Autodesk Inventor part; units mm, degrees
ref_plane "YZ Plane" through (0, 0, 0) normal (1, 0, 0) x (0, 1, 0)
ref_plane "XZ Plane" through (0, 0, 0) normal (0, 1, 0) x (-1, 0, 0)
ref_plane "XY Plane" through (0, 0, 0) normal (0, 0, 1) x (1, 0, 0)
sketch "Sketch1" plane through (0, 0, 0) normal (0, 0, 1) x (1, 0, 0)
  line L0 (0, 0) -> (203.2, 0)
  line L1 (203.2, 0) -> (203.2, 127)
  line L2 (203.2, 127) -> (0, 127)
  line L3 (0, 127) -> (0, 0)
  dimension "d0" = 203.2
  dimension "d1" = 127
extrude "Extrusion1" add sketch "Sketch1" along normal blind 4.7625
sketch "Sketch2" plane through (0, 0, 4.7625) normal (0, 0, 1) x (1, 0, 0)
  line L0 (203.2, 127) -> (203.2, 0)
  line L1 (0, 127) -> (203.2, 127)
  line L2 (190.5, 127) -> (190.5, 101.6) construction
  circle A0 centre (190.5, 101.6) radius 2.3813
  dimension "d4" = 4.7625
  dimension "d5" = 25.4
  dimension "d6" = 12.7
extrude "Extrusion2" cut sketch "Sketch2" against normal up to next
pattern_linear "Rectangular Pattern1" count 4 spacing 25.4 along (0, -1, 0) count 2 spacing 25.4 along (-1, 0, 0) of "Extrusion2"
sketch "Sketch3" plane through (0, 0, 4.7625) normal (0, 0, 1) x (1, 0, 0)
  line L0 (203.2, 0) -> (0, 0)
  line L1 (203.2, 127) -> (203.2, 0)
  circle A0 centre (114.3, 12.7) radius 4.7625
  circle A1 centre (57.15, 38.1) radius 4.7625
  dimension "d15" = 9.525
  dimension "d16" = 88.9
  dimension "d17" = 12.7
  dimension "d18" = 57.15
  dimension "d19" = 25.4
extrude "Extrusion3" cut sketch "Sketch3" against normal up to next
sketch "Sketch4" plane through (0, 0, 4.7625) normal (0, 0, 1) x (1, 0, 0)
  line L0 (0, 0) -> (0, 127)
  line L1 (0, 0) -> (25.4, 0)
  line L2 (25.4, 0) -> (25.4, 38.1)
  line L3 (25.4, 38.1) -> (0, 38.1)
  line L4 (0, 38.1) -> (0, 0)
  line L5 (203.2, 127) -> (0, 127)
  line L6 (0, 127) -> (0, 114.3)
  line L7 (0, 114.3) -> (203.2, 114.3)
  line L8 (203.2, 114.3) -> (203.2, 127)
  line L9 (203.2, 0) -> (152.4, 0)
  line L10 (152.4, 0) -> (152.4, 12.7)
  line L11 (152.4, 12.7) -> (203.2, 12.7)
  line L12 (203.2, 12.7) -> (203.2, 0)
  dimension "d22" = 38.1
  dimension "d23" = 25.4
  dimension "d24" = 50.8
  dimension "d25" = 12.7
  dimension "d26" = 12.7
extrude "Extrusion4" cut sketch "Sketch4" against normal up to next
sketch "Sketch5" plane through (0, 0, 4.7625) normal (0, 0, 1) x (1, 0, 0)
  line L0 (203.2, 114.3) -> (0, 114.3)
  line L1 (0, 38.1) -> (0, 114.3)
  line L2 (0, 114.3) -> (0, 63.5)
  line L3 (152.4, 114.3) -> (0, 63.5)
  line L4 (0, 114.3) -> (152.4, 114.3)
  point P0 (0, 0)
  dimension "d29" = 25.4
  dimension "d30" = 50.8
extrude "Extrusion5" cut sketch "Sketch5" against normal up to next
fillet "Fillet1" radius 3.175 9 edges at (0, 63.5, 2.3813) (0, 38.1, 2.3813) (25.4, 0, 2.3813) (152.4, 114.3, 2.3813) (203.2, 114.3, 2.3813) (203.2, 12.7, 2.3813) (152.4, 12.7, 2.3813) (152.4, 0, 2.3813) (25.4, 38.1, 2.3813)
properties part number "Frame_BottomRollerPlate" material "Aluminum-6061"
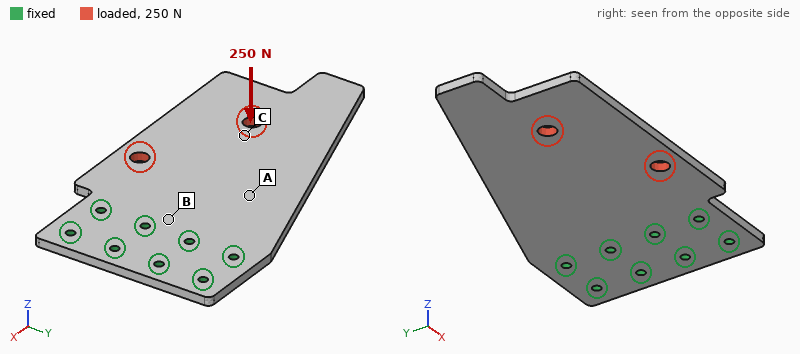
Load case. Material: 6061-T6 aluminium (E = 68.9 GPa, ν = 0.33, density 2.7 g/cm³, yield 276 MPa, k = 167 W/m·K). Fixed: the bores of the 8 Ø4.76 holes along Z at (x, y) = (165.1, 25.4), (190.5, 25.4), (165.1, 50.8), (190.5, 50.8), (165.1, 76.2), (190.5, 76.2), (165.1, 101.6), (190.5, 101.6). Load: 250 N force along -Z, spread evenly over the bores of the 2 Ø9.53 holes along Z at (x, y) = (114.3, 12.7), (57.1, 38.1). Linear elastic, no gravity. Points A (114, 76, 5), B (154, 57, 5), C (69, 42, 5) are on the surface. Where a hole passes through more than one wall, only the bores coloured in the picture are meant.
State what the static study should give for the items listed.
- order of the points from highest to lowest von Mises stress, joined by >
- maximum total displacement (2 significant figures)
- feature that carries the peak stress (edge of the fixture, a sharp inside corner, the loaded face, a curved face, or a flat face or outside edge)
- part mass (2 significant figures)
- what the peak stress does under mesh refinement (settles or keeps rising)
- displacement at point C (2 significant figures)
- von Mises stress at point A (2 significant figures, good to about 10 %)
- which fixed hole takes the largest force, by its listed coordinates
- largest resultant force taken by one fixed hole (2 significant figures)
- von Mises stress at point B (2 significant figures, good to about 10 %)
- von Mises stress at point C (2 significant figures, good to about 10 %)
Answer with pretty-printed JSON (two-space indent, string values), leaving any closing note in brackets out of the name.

{
  "order of the points from highest to lowest von Mises stress, joined by >": "B > A > C",
  "maximum total displacement": "1.9 mm",
  "feature that carries the peak stress": "edge of the fixture",
  "part mass": "220 g",
  "what the peak stress does under mesh refinement": "keeps rising",
  "displacement at point C": "0.94 mm",
  "von Mises stress at point A": "25 MPa",
  "which fixed hole takes the largest force, by its listed coordinates": "(165.1, 25.4)",
  "largest resultant force taken by one fixed hole": "240 N",
  "von Mises stress at point B": "43 MPa",
  "von Mises stress at point C": "8.5 MPa"
}
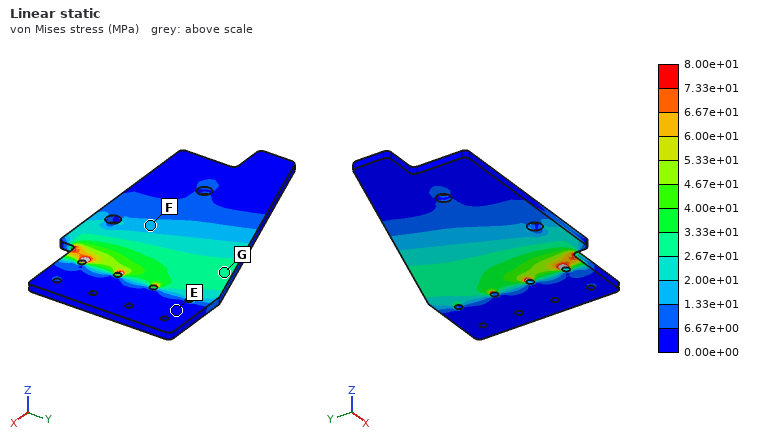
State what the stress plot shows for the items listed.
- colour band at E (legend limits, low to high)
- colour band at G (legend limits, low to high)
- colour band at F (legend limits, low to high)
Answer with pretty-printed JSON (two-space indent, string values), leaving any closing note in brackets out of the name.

{
  "colour band at E": "0.00e+00 to 6.67e+00 MPa",
  "colour band at G": "2.67e+01 to 3.33e+01 MPa",
  "colour band at F": "1.33e+01 to 2.00e+01 MPa"
}
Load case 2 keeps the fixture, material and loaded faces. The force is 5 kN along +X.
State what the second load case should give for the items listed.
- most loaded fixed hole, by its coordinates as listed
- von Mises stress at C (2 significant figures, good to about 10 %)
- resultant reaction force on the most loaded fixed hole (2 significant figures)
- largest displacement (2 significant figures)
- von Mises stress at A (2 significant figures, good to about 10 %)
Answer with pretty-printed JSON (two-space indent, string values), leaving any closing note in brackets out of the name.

{
  "most loaded fixed hole, by its coordinates as listed": "(165.1, 25.4)",
  "von Mises stress at C": "15 MPa",
  "resultant reaction force on the most loaded fixed hole": "3.1 kN",
  "largest displacement": "65 µm",
  "von Mises stress at A": "4.9 MPa"
}
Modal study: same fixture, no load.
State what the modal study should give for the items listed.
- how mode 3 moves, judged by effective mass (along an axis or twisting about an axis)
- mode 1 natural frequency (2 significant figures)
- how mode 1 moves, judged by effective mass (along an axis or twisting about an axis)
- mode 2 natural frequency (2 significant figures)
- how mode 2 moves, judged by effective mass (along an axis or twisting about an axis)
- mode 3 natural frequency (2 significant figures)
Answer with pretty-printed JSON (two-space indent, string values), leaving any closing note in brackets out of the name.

{
  "how mode 3 moves, judged by effective mass": "along Z",
  "mode 1 natural frequency": "190 Hz",
  "how mode 1 moves, judged by effective mass": "along Z",
  "mode 2 natural frequency": "750 Hz",
  "how mode 2 moves, judged by effective mass": "twisting about X",
  "mode 3 natural frequency": "1000 Hz"
}
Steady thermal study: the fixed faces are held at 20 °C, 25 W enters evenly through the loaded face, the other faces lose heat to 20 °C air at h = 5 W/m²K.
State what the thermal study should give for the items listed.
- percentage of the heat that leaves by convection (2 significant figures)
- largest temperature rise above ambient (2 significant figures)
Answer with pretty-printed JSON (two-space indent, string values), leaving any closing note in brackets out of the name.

{
  "percentage of the heat that leaves by convection": "9.7 %",
  "largest temperature rise above ambient": "29 K"
}
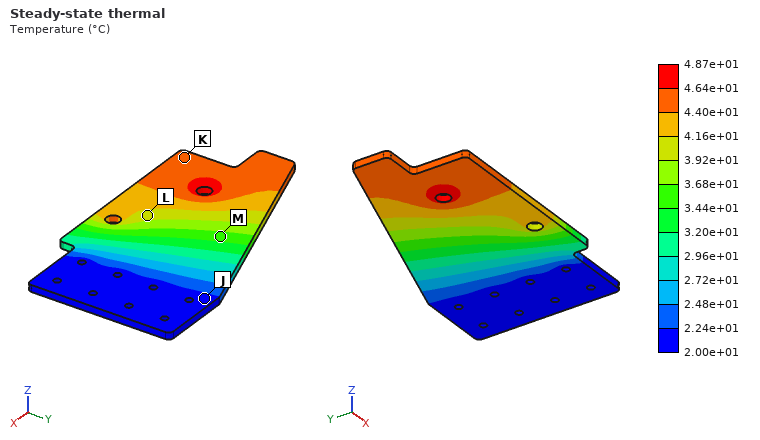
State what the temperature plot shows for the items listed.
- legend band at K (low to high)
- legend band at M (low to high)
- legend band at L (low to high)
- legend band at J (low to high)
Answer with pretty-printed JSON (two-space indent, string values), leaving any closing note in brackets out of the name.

{
  "legend band at K": "4.40e+01 to 4.64e+01 °C",
  "legend band at M": "3.44e+01 to 3.68e+01 °C",
  "legend band at L": "3.92e+01 to 4.16e+01 °C",
  "legend band at J": "2.00e+01 to 2.24e+01 °C"
}
